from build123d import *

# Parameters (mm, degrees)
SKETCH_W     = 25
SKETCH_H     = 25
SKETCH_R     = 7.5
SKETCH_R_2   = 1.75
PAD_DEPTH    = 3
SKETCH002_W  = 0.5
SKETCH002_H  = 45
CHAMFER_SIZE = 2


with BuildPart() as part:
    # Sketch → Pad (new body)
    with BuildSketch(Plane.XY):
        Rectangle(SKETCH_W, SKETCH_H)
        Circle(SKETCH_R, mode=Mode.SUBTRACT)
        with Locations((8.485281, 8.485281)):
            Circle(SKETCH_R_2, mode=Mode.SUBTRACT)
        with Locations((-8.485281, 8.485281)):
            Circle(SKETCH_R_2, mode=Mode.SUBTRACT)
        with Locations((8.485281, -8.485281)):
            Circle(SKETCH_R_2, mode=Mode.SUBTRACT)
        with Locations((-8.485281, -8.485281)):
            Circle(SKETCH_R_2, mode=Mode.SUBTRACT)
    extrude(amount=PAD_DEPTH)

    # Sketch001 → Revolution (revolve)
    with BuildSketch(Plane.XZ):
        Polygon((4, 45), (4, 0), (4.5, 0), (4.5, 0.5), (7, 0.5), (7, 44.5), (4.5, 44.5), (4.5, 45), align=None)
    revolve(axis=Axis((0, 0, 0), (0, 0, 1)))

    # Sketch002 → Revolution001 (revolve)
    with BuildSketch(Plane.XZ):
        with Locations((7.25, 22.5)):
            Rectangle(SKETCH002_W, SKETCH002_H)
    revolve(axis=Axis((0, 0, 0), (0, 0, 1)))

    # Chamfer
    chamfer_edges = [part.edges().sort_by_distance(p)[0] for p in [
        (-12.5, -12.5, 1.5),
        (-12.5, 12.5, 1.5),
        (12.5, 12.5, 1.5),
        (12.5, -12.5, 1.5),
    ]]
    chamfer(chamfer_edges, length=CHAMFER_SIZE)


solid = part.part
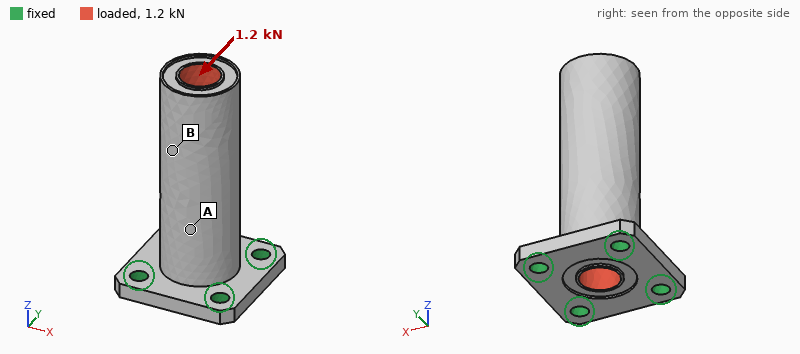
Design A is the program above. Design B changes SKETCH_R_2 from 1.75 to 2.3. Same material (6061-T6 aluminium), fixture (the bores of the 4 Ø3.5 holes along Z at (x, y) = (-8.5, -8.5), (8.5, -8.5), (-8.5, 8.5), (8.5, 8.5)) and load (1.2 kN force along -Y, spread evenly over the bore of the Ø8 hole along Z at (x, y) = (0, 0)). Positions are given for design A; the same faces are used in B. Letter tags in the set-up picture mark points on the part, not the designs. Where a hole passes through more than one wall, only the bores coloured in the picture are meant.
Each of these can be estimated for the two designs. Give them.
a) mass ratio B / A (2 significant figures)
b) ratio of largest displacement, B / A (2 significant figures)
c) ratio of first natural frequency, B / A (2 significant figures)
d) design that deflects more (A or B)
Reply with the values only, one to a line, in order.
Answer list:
0.99
0.90
1.1
A
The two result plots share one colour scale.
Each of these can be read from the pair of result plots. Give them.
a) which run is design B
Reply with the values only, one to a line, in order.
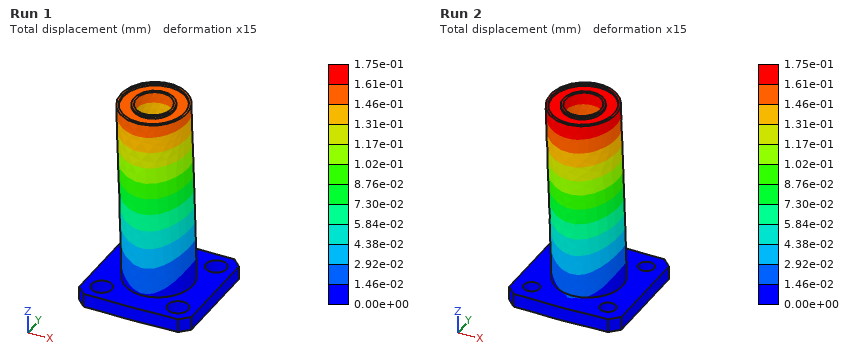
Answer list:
Run 1
